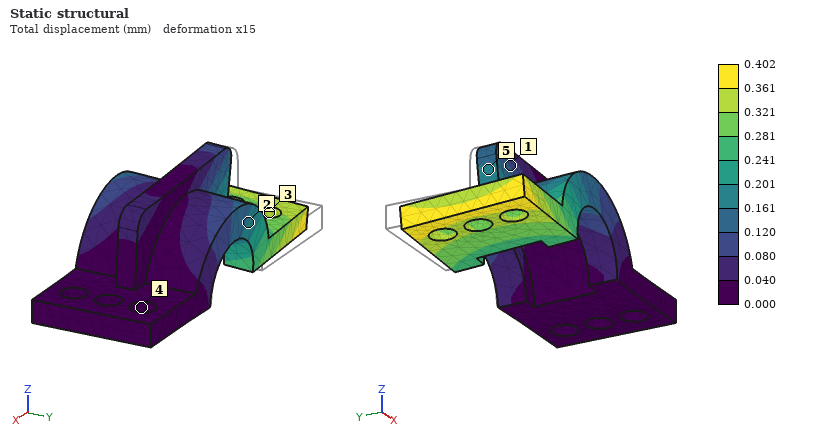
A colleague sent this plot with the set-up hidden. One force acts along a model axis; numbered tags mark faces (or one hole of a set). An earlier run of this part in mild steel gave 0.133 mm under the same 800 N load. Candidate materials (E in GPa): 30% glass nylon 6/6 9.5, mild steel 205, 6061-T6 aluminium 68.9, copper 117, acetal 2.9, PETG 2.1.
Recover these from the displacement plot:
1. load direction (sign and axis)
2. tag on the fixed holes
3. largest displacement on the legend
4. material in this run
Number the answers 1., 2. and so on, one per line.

1. -Y
2. 4
3. 0.402 mm
4. 6061-T6 aluminium
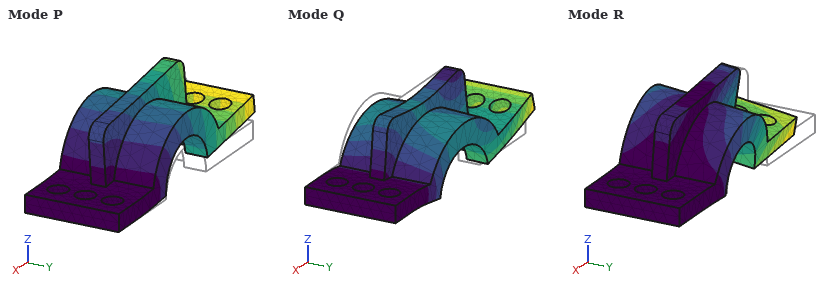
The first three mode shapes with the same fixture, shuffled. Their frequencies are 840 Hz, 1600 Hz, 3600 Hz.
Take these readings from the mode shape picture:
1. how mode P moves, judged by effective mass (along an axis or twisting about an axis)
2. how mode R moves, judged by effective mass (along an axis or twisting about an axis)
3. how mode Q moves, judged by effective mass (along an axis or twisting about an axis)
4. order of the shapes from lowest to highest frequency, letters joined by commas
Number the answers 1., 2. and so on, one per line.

1. along Z
2. along Y
3. along X
4. P, R, Q
